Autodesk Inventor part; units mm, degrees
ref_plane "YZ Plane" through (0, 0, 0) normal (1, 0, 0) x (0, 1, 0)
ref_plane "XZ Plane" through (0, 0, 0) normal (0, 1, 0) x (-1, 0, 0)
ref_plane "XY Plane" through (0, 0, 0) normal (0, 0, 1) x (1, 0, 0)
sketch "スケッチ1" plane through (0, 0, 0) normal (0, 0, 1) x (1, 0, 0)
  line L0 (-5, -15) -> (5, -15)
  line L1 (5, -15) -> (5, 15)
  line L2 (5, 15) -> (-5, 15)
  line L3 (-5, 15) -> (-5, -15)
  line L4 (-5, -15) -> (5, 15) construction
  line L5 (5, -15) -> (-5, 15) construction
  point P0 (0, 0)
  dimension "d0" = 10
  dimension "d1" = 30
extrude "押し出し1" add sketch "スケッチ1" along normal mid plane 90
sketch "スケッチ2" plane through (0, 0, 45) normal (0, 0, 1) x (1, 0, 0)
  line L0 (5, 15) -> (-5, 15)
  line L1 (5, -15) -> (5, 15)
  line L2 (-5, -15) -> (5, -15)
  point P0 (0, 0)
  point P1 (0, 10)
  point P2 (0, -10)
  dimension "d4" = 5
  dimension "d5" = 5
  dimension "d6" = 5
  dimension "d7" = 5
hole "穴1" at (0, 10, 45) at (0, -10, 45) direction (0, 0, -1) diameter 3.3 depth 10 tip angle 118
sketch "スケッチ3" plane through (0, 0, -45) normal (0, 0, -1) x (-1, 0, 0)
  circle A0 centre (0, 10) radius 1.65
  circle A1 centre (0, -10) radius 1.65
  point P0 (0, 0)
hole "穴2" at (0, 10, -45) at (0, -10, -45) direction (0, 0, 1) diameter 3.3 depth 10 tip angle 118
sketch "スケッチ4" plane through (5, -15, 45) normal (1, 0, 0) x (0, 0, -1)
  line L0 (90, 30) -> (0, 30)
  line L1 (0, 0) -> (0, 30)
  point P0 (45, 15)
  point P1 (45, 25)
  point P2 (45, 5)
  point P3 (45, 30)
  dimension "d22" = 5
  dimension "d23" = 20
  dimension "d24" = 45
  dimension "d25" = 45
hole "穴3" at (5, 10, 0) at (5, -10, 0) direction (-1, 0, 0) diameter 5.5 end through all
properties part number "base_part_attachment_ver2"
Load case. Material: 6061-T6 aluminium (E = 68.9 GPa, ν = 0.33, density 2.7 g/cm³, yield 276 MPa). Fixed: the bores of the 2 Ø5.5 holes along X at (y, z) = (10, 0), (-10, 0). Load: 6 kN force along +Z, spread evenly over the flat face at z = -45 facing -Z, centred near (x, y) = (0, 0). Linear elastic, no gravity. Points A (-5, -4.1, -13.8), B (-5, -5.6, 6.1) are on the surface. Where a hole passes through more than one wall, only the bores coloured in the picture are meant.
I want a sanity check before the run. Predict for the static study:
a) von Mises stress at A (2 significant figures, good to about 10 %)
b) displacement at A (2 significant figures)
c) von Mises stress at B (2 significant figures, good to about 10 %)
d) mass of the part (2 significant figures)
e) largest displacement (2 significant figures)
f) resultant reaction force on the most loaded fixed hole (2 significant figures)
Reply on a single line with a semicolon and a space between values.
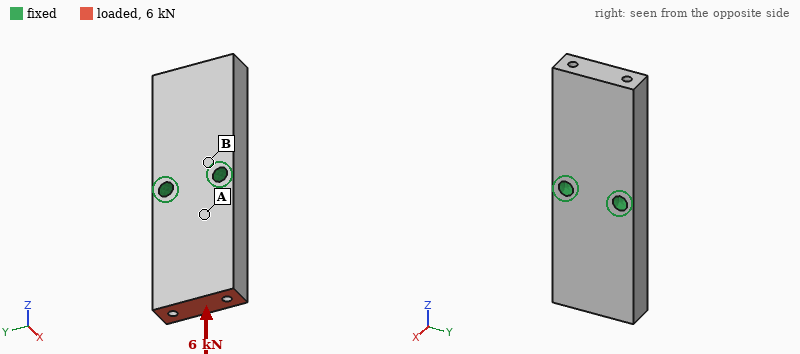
19 MPa; 4.0 µm; 5.7 MPa; 71 g; 13 µm; 3.0 kN
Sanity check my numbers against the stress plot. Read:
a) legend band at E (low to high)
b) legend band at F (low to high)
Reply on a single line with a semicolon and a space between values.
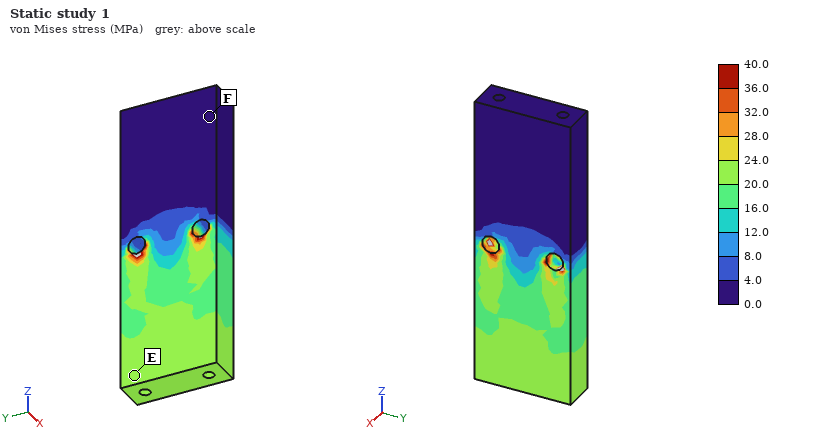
20.0 to 24.0 MPa; 0.0 to 4.0 MPa
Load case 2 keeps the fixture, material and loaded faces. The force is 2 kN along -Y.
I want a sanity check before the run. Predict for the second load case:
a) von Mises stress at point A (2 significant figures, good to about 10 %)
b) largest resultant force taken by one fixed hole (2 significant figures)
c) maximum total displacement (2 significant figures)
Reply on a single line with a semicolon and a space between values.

20 MPa; 4.1 kN; 55 µm
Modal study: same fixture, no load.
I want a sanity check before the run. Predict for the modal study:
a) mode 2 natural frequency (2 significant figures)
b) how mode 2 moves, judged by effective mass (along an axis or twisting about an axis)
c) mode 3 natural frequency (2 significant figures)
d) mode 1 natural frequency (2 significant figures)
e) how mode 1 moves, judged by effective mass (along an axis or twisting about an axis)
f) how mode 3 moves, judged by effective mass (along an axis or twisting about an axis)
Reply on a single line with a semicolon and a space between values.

4300 Hz; along X; 9900 Hz; 4000 Hz; twisting about Y; twisting about X
